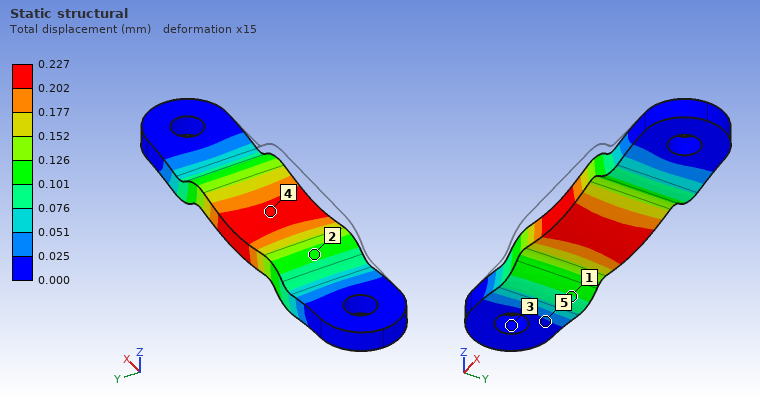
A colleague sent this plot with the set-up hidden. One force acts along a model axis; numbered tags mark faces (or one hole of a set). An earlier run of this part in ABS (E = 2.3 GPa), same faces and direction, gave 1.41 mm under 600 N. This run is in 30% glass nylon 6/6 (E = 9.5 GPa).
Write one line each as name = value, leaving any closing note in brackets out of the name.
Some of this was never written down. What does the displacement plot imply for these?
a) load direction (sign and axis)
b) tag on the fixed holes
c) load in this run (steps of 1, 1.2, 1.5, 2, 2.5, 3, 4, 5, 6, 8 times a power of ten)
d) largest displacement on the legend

load direction = -Z
tag on the fixed holes = 3
load in this run = 400 N
largest displacement on the legend = 0.227 mm
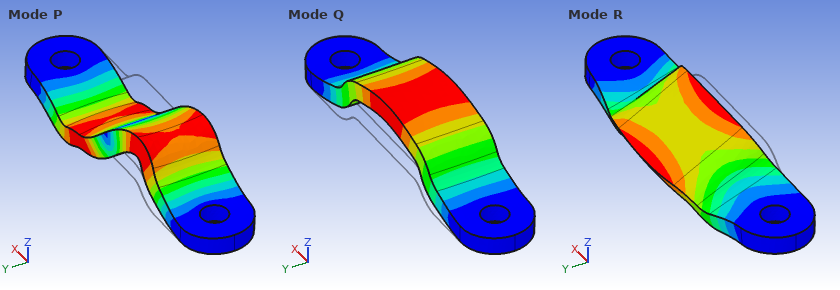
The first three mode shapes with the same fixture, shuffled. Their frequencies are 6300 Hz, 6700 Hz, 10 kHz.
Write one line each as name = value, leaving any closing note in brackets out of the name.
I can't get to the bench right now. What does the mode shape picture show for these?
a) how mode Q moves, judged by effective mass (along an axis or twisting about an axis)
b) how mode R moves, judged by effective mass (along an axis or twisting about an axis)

how mode Q moves, judged by effective mass = along Z
how mode R moves, judged by effective mass = along Y
